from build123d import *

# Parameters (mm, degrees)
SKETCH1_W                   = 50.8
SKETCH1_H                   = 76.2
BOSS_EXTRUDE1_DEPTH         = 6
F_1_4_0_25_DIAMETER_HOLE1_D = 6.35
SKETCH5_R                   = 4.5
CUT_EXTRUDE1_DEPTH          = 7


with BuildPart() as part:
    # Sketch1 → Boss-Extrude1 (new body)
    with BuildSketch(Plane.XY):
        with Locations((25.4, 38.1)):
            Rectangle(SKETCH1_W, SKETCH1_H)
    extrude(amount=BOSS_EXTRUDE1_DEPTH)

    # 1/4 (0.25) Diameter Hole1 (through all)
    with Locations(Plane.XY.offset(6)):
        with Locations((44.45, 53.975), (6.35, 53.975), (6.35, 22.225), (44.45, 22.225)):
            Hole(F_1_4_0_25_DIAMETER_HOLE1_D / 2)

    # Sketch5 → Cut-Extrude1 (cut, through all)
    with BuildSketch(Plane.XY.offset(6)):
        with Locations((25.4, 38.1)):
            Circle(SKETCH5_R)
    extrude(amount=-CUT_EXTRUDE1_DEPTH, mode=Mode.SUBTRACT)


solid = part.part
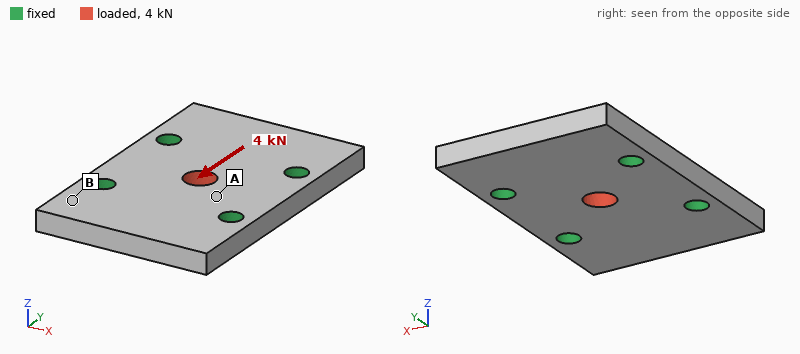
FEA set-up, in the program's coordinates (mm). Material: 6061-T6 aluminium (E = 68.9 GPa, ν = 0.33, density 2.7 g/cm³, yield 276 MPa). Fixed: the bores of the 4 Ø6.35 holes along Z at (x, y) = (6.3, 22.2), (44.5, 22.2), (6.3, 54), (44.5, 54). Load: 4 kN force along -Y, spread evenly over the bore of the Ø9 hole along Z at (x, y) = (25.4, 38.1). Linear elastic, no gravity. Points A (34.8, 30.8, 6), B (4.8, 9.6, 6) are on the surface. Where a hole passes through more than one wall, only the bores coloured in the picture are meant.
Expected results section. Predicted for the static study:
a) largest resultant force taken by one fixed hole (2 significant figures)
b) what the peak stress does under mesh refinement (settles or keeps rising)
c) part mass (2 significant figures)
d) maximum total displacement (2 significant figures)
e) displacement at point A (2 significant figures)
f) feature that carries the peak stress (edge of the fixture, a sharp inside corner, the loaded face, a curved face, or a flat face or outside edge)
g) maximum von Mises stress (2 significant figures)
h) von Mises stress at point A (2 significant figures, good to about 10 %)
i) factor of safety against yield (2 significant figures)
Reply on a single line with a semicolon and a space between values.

1.0 kN; settles; 60 g; 5.6 µm; 2.4 µm; the loaded face; 41 MPa; 14 MPa; 6.8
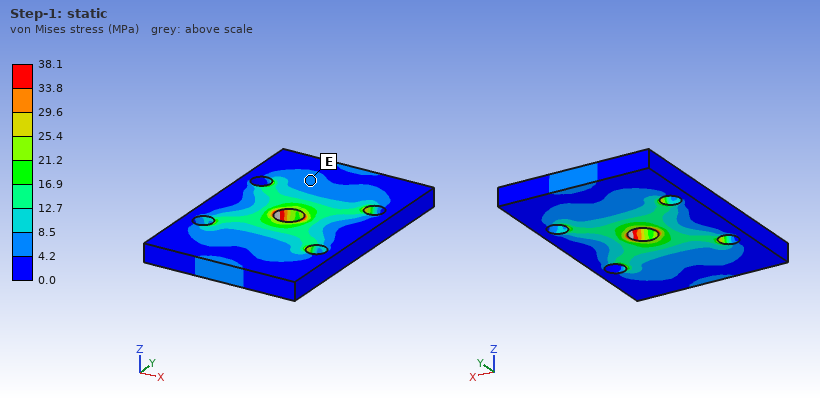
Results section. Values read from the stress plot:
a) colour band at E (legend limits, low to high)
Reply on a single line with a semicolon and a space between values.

4.2 to 8.5 MPa
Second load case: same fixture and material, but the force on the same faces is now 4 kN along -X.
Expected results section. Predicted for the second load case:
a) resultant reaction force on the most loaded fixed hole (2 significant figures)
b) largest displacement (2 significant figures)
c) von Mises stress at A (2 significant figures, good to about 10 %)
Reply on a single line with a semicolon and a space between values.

1.1 kN; 5.4 µm; 16 MPa
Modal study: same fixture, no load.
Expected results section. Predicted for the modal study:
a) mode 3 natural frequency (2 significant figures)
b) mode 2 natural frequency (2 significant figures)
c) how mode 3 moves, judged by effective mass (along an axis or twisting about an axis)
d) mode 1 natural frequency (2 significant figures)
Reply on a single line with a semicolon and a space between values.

14 kHz; 9100 Hz; twisting about Y; 9000 Hz
